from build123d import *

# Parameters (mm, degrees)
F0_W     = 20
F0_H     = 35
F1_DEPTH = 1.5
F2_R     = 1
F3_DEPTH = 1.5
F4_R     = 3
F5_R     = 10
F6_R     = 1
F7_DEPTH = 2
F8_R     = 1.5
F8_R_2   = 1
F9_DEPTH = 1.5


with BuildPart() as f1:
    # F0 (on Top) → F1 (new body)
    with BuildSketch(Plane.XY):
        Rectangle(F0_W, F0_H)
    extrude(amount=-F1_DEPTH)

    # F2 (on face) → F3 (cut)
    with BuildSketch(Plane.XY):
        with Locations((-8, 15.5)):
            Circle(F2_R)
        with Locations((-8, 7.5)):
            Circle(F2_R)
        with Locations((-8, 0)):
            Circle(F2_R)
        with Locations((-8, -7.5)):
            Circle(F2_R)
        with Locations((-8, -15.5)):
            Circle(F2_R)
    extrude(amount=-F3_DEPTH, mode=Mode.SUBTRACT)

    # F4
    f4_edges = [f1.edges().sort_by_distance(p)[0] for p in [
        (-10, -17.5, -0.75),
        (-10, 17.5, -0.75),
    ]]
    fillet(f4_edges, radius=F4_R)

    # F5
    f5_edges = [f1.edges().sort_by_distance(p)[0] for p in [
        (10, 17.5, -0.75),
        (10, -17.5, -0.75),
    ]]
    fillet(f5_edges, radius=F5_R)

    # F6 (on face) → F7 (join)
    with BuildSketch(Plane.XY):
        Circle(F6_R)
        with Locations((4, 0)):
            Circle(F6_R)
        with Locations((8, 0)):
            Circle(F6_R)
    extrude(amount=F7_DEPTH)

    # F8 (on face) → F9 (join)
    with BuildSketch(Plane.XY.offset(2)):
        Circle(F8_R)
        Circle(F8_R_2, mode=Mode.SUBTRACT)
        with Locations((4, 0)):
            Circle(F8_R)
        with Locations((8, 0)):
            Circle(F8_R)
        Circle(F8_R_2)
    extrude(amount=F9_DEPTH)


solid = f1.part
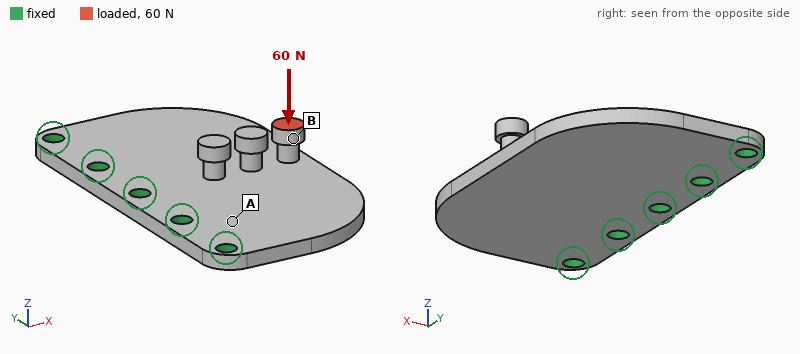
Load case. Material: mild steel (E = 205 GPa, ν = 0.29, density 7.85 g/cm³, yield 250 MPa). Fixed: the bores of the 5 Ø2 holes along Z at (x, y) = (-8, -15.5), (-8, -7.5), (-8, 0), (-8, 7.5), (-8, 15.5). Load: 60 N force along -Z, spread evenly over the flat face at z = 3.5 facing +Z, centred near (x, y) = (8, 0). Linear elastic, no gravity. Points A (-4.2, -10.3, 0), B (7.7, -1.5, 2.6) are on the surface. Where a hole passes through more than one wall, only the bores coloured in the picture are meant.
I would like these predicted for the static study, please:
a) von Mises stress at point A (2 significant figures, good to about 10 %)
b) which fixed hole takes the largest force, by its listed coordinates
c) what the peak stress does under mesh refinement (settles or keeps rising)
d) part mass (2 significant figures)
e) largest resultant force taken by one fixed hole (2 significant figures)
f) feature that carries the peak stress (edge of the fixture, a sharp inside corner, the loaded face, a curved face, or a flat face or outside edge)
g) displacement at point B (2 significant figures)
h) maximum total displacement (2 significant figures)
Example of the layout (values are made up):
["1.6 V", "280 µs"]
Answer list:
["50 MPa", "(-8, 0)", "keeps rising", "7.9 g", "25 N", "edge of the fixture", "46 µm", "55 µm"]
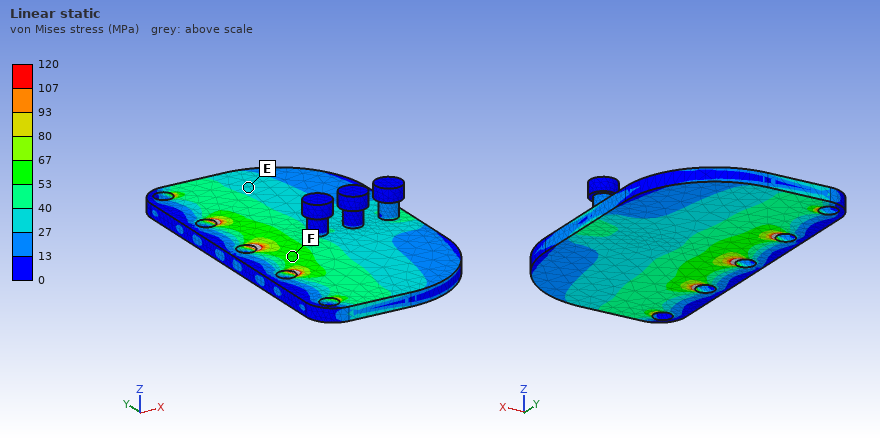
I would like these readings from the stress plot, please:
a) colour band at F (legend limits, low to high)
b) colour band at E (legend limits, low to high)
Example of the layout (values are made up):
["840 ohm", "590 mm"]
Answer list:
["53 to 67 MPa", "27 to 40 MPa"]
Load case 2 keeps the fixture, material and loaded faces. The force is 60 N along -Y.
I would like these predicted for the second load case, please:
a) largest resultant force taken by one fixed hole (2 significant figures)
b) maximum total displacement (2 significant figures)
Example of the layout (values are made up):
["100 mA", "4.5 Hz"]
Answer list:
["27 N", "18 µm"]
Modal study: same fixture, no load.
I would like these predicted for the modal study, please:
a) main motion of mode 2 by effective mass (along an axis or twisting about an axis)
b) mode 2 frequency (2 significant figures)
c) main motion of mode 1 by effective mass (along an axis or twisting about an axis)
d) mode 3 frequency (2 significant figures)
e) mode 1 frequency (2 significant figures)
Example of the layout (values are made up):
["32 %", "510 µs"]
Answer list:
["twisting about X", "7700 Hz", "along Z", "14 kHz", "4200 Hz"]
